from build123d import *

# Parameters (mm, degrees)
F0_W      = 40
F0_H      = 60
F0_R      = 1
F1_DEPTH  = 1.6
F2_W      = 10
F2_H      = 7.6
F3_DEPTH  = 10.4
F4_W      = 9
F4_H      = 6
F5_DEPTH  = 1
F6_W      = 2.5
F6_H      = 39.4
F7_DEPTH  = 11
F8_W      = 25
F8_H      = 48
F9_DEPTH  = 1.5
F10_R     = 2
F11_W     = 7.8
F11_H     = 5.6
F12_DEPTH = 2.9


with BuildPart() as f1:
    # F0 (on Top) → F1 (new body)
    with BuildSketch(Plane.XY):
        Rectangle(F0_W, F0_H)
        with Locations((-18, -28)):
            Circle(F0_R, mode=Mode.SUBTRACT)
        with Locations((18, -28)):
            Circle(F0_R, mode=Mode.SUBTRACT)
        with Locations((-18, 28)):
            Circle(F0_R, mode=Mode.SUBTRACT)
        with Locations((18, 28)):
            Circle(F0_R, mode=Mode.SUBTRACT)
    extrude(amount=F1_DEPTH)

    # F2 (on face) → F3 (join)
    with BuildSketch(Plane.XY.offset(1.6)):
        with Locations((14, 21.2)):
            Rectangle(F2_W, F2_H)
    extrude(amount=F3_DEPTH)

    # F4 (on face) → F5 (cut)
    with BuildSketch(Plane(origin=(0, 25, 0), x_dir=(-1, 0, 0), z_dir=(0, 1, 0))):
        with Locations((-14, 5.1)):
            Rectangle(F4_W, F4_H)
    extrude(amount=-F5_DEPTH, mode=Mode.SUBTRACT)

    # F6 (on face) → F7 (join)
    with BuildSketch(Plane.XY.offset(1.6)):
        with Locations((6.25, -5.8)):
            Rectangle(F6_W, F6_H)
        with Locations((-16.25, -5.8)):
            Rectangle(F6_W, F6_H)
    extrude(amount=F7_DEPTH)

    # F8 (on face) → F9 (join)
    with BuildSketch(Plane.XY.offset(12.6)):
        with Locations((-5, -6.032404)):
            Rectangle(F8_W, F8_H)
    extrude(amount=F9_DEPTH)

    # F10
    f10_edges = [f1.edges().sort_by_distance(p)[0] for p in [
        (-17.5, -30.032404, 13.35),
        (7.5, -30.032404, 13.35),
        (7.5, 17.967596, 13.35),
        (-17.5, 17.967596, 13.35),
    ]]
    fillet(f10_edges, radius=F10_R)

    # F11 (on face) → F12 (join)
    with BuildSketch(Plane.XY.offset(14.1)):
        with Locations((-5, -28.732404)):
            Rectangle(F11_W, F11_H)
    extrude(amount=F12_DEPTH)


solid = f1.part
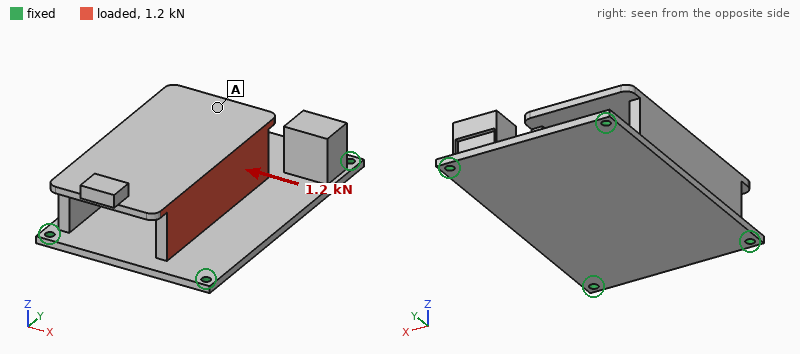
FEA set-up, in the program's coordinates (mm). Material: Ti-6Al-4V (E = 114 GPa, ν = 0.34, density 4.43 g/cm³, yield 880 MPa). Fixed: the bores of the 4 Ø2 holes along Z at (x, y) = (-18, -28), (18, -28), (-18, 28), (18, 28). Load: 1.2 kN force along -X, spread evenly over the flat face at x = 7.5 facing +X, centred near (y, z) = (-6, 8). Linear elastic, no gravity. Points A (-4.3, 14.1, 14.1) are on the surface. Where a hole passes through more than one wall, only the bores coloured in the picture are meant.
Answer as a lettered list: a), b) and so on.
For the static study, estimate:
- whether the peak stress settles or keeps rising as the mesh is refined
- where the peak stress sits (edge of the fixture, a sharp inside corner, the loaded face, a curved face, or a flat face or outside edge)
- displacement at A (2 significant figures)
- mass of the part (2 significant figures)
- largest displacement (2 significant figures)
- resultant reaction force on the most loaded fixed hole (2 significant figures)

a) keeps rising
b) edge of the fixture
c) 70 µm
d) 38 g
e) 92 µm
f) 500 N
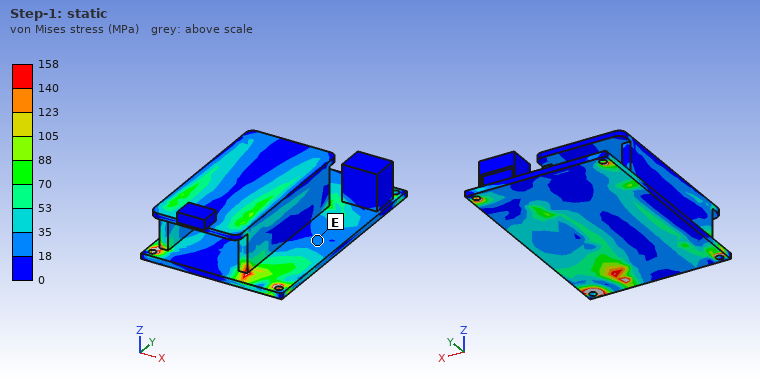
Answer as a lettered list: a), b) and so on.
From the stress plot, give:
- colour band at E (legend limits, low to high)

a) 18 to 35 MPa
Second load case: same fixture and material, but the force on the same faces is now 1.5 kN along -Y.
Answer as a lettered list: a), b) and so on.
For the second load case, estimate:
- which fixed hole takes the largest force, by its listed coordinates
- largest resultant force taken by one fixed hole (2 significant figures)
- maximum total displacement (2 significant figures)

a) (18, -28)
b) 480 N
c) 0.12 mm
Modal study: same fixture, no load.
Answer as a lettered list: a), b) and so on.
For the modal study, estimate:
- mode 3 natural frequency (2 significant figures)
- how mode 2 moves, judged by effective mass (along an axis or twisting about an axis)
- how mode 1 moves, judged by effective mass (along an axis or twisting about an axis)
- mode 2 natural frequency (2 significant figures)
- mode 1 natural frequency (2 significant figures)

a) 5300 Hz
b) along X
c) along Z
d) 3400 Hz
e) 2300 Hz
